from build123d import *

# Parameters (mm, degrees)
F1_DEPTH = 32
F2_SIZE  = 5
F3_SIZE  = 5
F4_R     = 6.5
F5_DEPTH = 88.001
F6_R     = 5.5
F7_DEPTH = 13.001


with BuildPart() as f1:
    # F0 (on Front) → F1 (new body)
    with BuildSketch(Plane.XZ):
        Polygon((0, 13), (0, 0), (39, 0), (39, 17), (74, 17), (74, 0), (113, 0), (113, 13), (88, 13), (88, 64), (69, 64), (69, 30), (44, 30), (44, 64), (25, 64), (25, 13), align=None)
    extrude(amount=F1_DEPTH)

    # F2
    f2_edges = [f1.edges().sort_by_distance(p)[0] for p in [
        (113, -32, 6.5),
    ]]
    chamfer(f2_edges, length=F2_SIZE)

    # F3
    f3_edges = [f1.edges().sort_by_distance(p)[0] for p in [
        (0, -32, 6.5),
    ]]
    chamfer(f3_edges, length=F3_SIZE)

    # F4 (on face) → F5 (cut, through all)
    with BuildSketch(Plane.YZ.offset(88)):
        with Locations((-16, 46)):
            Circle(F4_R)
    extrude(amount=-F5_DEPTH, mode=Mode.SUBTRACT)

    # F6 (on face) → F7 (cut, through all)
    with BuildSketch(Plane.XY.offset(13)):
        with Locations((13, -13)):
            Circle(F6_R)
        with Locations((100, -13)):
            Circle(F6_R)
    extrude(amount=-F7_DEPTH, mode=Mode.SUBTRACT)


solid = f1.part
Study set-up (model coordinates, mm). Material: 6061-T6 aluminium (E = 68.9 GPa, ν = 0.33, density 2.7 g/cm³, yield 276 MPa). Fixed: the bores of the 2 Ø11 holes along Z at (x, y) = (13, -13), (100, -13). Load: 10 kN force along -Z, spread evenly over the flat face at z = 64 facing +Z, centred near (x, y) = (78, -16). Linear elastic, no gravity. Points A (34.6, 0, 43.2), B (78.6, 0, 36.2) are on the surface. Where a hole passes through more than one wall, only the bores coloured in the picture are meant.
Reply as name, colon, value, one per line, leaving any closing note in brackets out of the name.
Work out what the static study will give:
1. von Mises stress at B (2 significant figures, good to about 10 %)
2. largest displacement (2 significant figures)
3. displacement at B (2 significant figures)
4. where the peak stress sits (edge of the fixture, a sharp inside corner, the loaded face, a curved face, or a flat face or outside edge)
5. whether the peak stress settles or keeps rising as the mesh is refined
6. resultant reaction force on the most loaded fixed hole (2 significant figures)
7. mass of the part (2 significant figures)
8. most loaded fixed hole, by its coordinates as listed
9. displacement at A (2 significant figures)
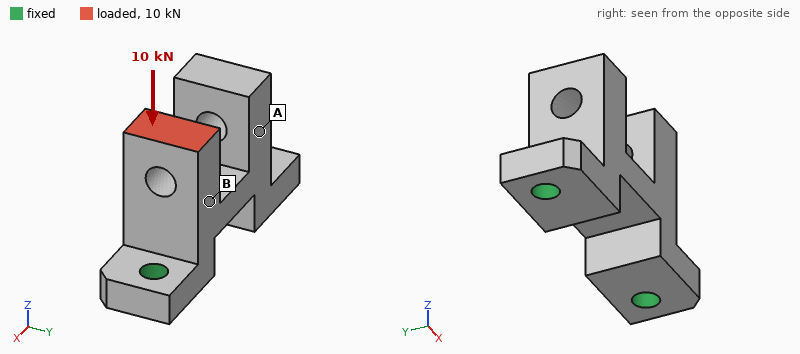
von Mises stress at B: 23 MPa
largest displacement: 49 µm
displacement at B: 28 µm
where the peak stress sits: edge of the fixture
whether the peak stress settles or keeps rising as the mesh is refined: keeps rising
resultant reaction force on the most loaded fixed hole: 9.0 kN
mass of the part: 260 g
most loaded fixed hole, by its coordinates as listed: (100, -13)
displacement at A: 10 µm
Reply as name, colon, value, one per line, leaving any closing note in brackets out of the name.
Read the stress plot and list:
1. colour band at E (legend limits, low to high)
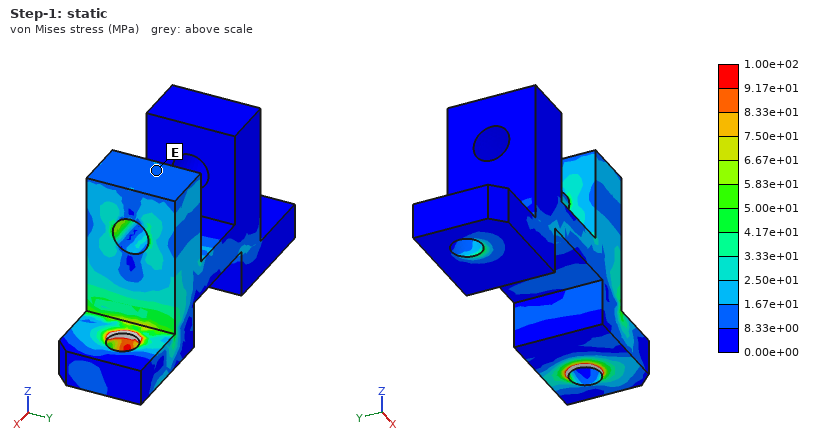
colour band at E: 8.33e+00 to 1.67e+01 MPa
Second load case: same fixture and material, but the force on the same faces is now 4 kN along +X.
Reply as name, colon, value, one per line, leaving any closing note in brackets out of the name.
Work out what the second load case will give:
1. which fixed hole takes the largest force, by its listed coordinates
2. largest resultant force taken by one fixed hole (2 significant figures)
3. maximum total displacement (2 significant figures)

which fixed hole takes the largest force, by its listed coordinates: (13, -13)
largest resultant force taken by one fixed hole: 6.1 kN
maximum total displacement: 0.17 mm
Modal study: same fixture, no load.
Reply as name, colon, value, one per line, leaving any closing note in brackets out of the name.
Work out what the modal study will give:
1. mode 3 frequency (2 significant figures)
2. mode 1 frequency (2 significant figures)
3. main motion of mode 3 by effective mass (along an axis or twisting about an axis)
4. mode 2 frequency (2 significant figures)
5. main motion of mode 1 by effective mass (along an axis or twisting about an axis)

mode 3 frequency: 5400 Hz
mode 1 frequency: 2700 Hz
main motion of mode 3 by effective mass: along X
mode 2 frequency: 4500 Hz
main motion of mode 1 by effective mass: along Y
